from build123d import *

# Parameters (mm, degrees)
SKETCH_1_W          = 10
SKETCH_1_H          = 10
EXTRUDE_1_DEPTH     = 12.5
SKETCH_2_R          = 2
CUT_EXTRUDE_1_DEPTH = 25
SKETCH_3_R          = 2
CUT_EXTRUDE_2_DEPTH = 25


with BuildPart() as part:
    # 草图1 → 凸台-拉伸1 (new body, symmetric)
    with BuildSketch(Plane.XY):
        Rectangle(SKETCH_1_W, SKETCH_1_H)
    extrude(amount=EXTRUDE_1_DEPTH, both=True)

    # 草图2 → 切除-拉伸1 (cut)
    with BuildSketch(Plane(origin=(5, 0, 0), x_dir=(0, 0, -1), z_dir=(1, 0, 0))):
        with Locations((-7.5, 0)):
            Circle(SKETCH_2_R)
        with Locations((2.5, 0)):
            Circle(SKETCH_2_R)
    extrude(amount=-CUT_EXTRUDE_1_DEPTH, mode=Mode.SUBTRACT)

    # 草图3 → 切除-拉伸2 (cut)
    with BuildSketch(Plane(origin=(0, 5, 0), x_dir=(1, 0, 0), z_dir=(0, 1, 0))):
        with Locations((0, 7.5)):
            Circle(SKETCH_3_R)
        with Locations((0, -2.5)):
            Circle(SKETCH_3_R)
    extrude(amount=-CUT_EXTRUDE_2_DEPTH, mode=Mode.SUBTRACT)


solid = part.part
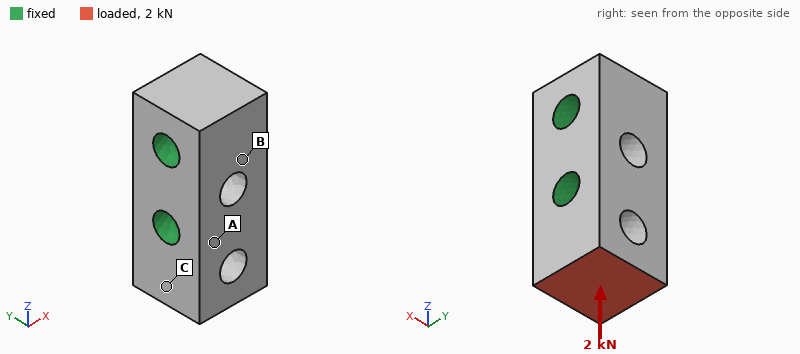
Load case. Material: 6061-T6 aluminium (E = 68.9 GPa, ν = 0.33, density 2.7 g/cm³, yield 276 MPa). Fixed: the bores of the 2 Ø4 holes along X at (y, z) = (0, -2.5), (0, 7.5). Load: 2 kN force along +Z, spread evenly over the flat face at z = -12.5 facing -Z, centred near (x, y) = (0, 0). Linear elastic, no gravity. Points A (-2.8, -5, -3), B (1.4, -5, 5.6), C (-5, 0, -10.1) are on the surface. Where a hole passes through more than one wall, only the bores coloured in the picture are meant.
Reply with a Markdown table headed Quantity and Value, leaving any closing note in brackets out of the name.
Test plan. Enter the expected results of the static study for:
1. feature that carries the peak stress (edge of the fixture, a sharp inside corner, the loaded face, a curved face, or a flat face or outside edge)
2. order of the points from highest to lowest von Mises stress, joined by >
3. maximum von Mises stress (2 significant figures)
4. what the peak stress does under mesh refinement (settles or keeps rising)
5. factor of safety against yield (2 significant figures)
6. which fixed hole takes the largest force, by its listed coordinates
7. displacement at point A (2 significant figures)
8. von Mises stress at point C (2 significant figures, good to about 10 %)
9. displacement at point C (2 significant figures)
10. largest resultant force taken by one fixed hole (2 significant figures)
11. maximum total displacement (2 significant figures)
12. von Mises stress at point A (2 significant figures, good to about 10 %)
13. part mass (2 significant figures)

| Quantity | Value |
|---|---|
| feature that carries the peak stress | a curved face |
| order of the points from highest to lowest von Mises stress, joined by > | C > A > B |
| maximum von Mises stress | 83 MPa |
| what the peak stress does under mesh refinement | settles |
| factor of safety against yield | 3.3 |
| which fixed hole takes the largest force, by its listed coordinates | (0, -2.5) |
| displacement at point A | 0.90 µm |
| von Mises stress at point C | 22 MPa |
| displacement at point C | 2.6 µm |
| largest resultant force taken by one fixed hole | 1.9 kN |
| maximum total displacement | 5.1 µm |
| von Mises stress at point A | 14 MPa |
| part mass | 5.4 g |
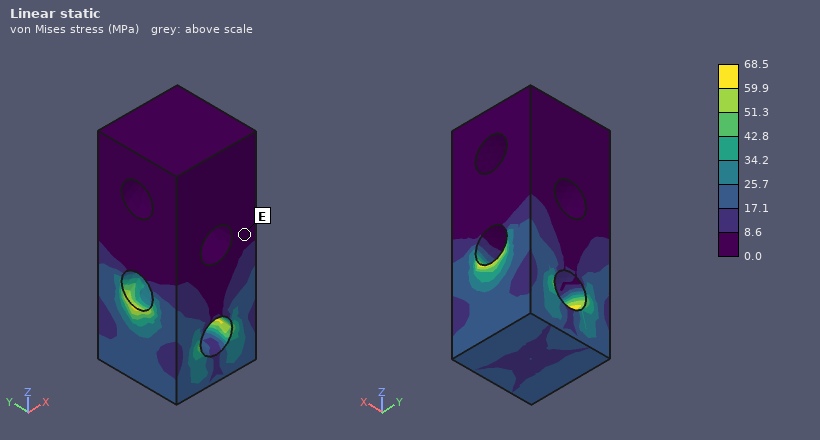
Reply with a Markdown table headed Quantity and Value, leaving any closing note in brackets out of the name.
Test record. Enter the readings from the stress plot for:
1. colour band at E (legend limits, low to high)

| Quantity | Value |
|---|---|
| colour band at E | 0.0 to 8.6 MPa |
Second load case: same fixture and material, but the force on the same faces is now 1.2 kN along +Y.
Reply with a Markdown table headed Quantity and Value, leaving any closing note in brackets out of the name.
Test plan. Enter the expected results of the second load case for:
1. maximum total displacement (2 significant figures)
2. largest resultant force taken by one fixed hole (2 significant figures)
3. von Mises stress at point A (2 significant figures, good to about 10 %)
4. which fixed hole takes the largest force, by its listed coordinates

| Quantity | Value |
|---|---|
| maximum total displacement | 22 µm |
| largest resultant force taken by one fixed hole | 1.5 kN |
| von Mises stress at point A | 53 MPa |
| which fixed hole takes the largest force, by its listed coordinates | (0, -2.5) |
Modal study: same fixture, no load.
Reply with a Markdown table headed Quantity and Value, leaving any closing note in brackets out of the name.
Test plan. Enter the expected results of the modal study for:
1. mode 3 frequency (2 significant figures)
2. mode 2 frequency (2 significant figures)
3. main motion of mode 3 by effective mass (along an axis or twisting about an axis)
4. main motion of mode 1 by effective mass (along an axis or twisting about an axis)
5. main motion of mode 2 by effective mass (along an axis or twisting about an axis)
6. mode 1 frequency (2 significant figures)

| Quantity | Value |
|---|---|
| mode 3 frequency | 67 kHz |
| mode 2 frequency | 49 kHz |
| main motion of mode 3 by effective mass | twisting about Z |
| main motion of mode 1 by effective mass | along Y |
| main motion of mode 2 by effective mass | along X |
| mode 1 frequency | 45 kHz |
